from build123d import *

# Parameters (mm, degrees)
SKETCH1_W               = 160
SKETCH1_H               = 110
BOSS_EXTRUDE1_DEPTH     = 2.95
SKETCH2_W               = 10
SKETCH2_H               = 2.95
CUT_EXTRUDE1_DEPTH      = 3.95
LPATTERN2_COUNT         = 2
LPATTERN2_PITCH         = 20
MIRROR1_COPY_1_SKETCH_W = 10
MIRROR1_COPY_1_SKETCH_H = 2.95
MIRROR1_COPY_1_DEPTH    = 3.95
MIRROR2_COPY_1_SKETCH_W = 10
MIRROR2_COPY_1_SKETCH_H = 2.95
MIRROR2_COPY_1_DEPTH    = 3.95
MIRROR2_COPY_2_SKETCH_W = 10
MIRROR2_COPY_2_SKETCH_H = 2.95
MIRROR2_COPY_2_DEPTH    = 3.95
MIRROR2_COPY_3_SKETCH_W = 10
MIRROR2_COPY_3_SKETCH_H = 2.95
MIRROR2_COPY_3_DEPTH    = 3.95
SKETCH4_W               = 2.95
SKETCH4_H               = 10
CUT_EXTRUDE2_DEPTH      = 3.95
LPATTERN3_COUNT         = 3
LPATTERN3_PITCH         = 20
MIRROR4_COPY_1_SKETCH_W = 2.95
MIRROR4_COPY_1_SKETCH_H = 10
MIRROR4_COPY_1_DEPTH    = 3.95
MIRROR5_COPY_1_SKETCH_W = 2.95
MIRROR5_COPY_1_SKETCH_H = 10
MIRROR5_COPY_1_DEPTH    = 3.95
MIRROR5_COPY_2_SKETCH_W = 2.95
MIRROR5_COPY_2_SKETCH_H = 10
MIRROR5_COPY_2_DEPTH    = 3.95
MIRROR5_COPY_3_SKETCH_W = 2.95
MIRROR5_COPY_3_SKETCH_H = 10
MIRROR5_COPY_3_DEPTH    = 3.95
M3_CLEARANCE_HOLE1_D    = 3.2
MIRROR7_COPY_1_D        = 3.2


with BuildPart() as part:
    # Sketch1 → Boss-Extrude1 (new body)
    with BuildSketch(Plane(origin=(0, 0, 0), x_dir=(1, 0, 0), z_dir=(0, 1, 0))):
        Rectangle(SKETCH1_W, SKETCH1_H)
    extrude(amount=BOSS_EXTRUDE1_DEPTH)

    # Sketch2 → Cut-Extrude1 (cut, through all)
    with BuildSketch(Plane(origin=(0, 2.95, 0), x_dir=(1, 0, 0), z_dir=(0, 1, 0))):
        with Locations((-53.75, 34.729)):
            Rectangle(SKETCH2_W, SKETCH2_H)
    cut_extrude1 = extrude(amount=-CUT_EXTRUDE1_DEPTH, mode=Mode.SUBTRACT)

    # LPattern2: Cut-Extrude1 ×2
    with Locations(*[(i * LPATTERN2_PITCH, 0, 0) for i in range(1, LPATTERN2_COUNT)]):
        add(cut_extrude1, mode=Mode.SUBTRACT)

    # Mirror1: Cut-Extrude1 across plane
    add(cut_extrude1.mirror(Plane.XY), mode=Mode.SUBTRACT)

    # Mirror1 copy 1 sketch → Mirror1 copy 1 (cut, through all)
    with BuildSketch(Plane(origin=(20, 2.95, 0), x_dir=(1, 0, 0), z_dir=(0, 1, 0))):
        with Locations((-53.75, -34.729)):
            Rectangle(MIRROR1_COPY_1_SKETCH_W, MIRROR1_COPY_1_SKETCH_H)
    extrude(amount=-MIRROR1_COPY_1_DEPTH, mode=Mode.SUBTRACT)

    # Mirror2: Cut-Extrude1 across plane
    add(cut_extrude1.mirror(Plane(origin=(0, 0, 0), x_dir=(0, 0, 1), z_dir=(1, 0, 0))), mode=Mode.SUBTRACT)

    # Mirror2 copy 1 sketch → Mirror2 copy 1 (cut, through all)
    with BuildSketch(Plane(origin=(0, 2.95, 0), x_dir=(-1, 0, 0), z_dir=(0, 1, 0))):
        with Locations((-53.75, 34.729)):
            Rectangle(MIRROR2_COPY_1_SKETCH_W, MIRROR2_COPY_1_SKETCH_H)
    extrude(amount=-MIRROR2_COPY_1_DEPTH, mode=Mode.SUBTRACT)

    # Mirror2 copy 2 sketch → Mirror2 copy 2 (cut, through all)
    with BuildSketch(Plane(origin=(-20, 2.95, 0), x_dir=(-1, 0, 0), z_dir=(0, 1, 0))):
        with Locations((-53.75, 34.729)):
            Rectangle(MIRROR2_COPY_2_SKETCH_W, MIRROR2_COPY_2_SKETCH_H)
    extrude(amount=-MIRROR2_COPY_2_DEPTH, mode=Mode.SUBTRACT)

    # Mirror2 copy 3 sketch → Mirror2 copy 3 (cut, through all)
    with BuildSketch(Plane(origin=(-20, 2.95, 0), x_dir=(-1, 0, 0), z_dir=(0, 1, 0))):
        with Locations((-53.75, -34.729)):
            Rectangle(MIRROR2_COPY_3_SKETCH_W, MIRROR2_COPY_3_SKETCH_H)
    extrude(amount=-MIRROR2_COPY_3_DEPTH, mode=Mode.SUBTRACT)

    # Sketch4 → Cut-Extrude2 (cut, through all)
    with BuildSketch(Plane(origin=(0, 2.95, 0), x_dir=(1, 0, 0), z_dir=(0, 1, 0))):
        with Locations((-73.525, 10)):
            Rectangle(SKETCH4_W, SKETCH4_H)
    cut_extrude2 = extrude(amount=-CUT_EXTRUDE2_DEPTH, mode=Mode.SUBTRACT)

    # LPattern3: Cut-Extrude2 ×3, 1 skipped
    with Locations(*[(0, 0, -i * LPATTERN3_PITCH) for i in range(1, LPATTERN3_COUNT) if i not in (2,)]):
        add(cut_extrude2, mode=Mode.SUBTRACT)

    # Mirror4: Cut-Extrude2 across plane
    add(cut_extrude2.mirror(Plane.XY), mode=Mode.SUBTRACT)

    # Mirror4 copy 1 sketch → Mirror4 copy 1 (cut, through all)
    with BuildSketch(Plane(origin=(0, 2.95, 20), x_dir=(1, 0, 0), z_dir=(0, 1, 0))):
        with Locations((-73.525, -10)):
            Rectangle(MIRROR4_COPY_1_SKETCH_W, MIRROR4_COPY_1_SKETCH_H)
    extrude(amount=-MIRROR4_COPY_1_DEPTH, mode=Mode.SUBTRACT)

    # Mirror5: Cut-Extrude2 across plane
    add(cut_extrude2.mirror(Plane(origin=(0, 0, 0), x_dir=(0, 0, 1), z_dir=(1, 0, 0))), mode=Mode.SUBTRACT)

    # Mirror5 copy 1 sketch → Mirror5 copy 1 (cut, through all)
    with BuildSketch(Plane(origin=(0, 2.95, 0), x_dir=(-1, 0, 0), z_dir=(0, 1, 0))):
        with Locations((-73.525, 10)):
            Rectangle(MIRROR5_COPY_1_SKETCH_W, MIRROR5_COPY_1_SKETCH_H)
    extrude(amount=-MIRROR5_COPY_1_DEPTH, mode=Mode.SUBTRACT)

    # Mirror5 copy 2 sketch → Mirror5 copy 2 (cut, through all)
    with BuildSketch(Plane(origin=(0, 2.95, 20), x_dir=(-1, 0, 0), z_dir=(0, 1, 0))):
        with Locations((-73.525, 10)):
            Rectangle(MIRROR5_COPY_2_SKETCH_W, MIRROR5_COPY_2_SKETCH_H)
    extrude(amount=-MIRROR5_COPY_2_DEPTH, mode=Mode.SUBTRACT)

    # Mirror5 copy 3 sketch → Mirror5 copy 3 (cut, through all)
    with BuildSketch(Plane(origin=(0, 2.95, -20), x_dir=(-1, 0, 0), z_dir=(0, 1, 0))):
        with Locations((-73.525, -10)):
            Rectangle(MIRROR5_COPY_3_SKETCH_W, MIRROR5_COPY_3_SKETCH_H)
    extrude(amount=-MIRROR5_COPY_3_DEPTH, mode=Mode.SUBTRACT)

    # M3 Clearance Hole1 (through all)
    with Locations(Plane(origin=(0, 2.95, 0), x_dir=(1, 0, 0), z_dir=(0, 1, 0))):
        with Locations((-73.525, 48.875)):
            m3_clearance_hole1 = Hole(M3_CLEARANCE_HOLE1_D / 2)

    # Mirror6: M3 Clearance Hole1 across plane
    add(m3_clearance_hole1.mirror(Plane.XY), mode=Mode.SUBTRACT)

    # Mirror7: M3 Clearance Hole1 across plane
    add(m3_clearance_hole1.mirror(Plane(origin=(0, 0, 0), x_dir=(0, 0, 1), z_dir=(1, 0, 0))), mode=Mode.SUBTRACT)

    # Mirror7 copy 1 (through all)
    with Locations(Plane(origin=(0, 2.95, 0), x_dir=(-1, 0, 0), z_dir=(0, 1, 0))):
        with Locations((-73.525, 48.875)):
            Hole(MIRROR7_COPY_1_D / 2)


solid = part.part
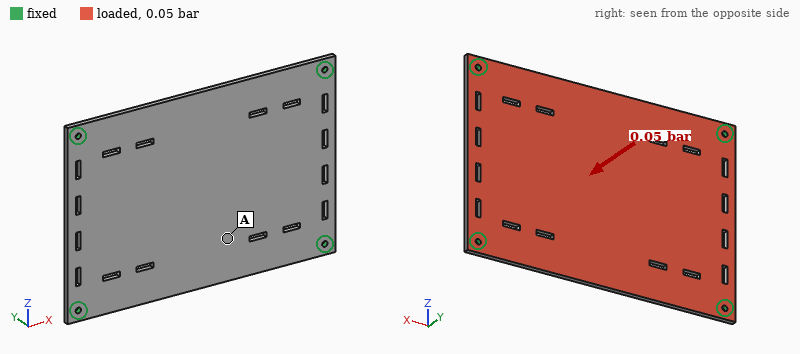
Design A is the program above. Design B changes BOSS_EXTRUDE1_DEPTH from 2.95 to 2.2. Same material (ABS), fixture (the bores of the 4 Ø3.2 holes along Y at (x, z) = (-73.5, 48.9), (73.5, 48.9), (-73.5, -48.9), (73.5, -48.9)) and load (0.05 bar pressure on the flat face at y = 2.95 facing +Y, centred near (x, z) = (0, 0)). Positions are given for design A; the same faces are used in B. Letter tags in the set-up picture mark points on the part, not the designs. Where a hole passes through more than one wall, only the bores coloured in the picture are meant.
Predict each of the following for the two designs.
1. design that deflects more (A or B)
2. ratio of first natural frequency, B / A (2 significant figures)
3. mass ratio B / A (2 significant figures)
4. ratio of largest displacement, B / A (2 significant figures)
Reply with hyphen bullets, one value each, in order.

- B
- 0.76
- 0.75
- 2.4
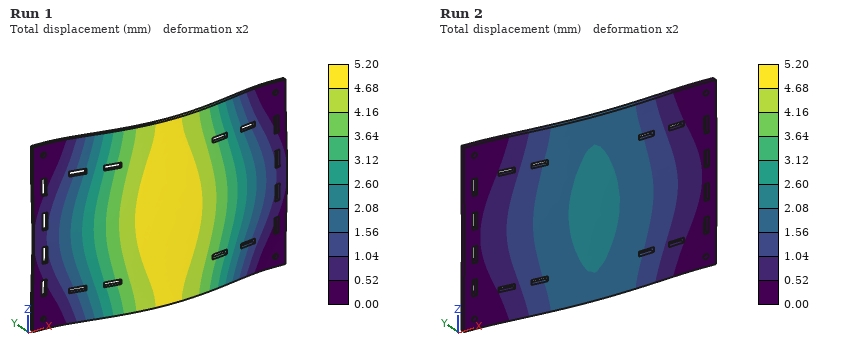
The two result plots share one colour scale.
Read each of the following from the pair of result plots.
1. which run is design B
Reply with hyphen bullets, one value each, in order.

- Run 1
